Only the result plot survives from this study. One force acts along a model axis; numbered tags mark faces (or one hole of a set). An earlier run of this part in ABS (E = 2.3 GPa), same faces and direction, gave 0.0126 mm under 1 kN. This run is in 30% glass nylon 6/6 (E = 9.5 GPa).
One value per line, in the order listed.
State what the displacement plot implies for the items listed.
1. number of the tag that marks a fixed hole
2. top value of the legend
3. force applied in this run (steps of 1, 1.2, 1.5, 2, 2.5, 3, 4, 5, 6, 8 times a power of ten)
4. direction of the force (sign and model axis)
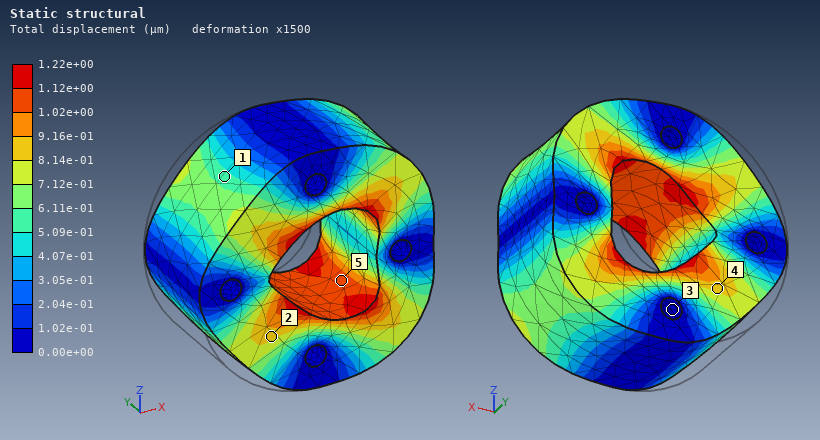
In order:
3
1.22e+00 µm
400 N
+X
